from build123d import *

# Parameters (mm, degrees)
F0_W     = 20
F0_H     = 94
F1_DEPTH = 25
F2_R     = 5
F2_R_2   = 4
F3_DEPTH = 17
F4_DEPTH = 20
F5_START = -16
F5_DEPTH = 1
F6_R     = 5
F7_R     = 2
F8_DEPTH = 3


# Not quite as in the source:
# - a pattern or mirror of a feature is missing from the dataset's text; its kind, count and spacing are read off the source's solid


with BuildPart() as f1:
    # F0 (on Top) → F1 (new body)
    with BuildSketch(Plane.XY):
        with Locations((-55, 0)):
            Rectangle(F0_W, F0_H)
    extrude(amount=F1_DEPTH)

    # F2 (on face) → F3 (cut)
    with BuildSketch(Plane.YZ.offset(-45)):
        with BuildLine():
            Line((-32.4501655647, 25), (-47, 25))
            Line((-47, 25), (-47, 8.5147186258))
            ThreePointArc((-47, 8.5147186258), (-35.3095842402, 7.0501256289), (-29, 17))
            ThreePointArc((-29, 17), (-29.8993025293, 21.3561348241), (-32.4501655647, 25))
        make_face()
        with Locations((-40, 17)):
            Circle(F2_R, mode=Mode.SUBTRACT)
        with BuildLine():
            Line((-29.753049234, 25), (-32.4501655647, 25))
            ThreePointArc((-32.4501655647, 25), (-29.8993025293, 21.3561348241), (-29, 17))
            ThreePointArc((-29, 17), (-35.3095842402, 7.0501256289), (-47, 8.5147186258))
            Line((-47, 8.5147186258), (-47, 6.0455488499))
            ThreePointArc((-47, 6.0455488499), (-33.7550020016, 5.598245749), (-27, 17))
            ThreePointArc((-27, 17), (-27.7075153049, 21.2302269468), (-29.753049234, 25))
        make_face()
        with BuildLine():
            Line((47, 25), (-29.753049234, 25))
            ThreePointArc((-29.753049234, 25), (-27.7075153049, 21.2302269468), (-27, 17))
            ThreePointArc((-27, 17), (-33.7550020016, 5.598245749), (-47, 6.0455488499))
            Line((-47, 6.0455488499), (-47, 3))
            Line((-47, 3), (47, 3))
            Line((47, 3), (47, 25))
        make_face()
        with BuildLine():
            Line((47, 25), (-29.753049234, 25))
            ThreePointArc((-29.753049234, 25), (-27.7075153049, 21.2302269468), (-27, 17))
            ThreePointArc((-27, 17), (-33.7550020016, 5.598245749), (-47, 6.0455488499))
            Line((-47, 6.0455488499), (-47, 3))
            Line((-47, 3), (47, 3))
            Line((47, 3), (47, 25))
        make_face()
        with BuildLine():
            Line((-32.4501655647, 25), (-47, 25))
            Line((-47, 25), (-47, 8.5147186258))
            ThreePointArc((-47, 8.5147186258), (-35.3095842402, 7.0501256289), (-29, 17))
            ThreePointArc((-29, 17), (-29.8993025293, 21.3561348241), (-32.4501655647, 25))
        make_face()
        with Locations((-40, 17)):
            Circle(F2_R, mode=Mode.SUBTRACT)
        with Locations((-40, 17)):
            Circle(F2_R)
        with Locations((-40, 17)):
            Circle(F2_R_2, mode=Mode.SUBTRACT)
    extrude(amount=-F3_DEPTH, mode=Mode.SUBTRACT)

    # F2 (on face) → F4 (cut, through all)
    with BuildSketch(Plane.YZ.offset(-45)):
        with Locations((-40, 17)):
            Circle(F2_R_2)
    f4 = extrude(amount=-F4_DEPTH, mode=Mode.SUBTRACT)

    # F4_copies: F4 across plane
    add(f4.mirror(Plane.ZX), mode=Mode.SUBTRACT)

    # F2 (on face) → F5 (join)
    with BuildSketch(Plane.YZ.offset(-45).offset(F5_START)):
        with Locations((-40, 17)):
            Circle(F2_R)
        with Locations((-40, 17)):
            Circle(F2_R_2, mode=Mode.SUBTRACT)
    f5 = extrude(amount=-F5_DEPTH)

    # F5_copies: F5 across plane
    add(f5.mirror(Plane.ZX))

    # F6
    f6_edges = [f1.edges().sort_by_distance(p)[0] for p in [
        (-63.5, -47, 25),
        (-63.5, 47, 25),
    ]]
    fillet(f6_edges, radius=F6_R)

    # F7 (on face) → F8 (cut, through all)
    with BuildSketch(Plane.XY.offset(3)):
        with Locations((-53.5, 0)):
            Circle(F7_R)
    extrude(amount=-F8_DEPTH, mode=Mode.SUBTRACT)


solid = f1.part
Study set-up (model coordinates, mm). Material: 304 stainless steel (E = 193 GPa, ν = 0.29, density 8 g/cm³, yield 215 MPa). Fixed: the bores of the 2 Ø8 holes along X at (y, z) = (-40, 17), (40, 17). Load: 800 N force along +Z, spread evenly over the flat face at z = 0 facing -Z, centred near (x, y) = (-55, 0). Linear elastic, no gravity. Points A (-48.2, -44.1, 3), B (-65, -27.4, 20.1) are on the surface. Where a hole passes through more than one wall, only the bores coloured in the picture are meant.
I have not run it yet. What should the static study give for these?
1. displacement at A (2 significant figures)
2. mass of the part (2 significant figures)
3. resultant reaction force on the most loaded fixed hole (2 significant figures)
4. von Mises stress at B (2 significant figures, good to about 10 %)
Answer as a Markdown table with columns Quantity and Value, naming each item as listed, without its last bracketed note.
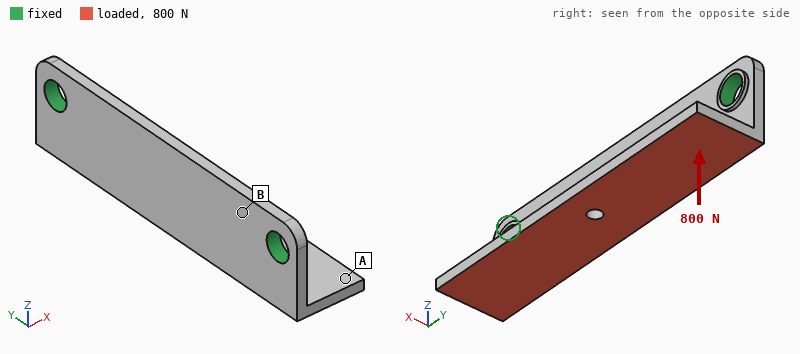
| Quantity | Value |
|---|---|
| displacement at A | 55 µm |
| mass of the part | 92 g |
| resultant reaction force on the most loaded fixed hole | 420 N |
| von Mises stress at B | 27 MPa |
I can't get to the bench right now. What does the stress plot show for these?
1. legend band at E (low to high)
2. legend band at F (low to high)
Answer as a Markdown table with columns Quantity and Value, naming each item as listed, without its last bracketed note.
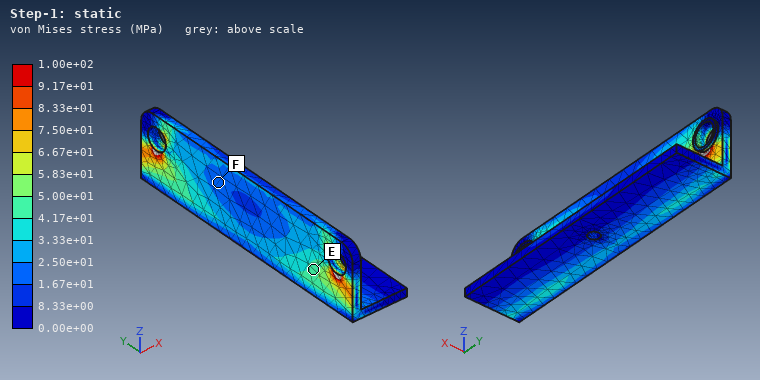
| Quantity | Value |
|---|---|
| legend band at E | 4.17e+01 to 5.00e+01 MPa |
| legend band at F | 1.67e+01 to 2.50e+01 MPa |
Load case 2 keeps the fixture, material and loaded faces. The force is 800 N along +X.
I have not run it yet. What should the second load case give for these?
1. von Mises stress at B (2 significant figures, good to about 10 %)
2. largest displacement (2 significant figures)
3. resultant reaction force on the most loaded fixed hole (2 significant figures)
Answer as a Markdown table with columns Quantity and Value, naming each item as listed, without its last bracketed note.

| Quantity | Value |
|---|---|
| von Mises stress at B | 38 MPa |
| largest displacement | 74 µm |
| resultant reaction force on the most loaded fixed hole | 420 N |
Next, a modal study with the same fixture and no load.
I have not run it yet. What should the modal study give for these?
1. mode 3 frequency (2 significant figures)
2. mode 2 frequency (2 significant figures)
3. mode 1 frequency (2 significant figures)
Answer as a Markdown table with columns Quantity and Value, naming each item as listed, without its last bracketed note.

| Quantity | Value |
|---|---|
| mode 3 frequency | 4000 Hz |
| mode 2 frequency | 3900 Hz |
| mode 1 frequency | 2500 Hz |
